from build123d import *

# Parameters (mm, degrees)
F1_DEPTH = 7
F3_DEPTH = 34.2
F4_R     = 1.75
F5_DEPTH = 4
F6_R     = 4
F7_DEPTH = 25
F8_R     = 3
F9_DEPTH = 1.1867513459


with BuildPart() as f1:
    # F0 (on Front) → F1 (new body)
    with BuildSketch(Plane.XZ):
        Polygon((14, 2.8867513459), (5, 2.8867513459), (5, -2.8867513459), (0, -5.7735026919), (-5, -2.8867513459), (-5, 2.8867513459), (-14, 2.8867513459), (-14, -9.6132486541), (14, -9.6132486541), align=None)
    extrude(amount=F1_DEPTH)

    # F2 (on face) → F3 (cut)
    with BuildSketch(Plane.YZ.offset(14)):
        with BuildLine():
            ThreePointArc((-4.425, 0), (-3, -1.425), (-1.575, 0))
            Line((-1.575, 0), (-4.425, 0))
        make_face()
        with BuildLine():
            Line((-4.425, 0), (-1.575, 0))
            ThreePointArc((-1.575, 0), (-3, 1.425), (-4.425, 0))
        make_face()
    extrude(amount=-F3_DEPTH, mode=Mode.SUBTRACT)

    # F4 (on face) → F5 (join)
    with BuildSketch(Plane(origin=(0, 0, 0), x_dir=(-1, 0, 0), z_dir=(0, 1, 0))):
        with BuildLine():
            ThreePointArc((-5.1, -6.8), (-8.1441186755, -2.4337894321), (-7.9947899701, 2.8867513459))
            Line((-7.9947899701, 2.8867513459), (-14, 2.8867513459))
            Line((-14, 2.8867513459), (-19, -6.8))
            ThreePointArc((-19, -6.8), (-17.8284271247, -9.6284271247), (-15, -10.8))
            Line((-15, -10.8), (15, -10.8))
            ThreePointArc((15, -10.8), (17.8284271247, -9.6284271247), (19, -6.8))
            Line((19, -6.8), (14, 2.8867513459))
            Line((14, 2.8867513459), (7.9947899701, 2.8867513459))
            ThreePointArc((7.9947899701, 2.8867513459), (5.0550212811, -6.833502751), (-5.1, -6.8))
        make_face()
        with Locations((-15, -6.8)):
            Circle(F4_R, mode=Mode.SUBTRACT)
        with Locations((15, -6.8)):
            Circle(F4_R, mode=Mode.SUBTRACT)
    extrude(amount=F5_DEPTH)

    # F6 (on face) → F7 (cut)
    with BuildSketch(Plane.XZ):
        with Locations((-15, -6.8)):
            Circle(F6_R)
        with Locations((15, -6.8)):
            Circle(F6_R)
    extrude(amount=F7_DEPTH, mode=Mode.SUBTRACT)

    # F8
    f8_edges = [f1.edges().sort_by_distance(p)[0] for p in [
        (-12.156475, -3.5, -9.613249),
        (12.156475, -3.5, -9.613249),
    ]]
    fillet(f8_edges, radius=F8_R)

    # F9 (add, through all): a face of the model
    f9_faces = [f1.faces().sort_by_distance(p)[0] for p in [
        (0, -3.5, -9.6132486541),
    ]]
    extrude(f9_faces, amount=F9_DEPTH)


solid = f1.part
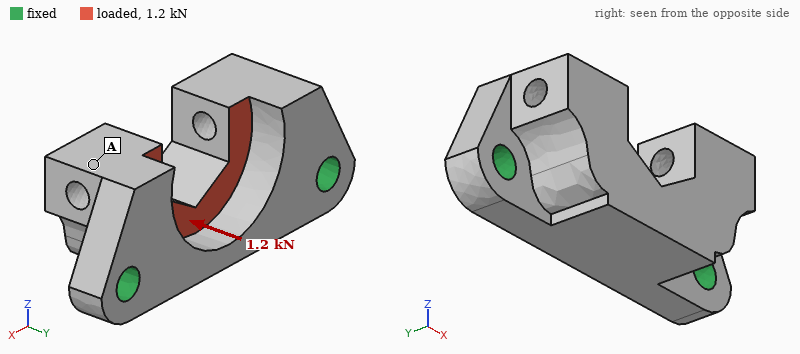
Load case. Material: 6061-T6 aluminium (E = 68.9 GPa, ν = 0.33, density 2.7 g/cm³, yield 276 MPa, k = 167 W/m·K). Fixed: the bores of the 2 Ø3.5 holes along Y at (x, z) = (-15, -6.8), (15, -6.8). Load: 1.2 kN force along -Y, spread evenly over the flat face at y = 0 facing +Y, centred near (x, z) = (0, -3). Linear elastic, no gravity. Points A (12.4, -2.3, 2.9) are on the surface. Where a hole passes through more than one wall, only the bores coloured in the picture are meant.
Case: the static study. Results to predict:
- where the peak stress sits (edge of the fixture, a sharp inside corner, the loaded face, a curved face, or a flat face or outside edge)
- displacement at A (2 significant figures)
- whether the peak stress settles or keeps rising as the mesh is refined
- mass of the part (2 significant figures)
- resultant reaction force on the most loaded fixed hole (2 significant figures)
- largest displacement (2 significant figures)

edge of the fixture
18 µm
keeps rising
7.6 g
740 N
29 µm
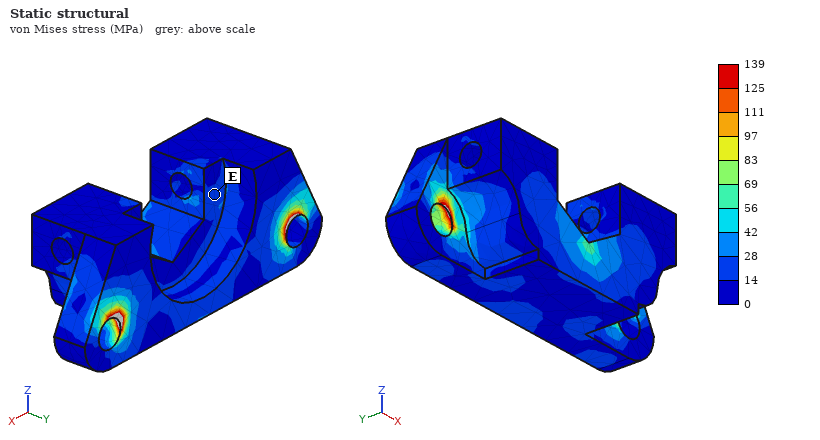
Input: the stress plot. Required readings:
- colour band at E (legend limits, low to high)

14 to 28 MPa
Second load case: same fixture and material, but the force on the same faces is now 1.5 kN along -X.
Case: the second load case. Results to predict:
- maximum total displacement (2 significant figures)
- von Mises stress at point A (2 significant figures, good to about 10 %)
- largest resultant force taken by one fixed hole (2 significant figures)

9.5 µm
7.4 MPa
770 N
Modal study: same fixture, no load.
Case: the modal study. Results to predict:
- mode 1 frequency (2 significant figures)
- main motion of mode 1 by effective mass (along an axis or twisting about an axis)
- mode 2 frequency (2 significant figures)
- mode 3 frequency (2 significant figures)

14 kHz
along Z
22 kHz
23 kHz
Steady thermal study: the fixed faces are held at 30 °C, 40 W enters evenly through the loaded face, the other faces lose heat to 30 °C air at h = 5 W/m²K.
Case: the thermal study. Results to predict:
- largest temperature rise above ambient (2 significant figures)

26 K
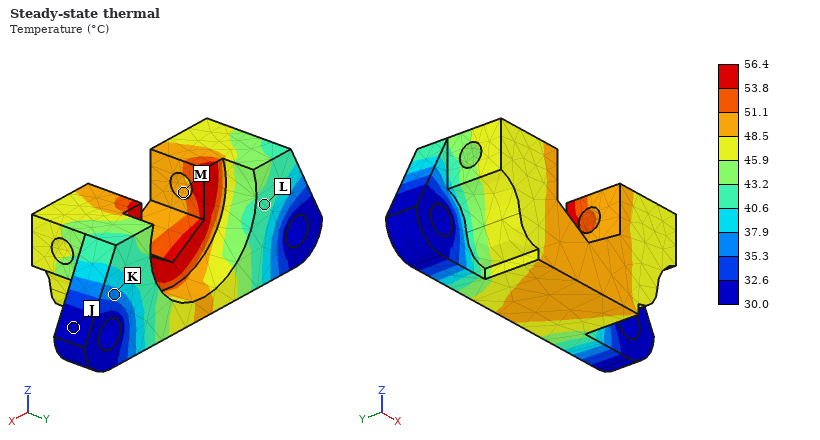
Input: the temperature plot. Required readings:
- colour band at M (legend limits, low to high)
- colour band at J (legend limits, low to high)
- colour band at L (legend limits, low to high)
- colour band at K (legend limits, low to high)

48.5 to 51.1 °C
30.0 to 32.6 °C
40.6 to 43.2 °C
35.3 to 37.9 °C
